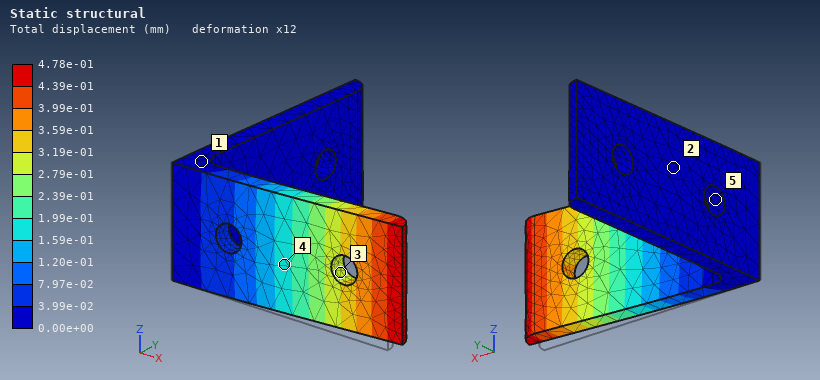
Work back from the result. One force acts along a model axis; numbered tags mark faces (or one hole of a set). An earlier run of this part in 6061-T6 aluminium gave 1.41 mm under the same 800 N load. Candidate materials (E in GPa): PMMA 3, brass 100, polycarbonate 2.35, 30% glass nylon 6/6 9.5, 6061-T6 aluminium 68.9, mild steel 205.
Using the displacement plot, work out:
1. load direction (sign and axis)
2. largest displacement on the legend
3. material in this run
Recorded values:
+Y
4.78e-01 mm
mild steel
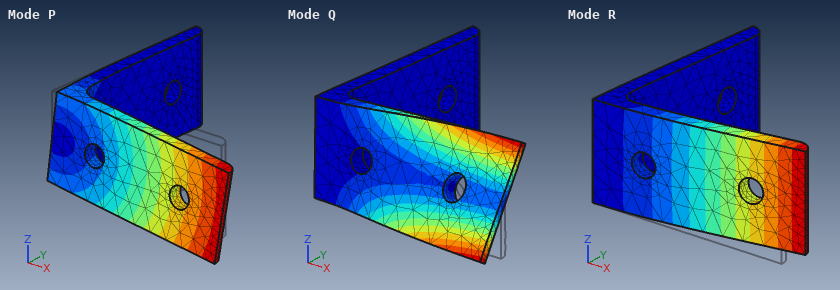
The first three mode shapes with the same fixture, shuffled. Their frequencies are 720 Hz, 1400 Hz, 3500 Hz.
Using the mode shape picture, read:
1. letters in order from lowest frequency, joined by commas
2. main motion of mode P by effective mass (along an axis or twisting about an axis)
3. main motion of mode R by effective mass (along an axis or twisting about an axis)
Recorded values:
R, P, Q
along Z
along Y
